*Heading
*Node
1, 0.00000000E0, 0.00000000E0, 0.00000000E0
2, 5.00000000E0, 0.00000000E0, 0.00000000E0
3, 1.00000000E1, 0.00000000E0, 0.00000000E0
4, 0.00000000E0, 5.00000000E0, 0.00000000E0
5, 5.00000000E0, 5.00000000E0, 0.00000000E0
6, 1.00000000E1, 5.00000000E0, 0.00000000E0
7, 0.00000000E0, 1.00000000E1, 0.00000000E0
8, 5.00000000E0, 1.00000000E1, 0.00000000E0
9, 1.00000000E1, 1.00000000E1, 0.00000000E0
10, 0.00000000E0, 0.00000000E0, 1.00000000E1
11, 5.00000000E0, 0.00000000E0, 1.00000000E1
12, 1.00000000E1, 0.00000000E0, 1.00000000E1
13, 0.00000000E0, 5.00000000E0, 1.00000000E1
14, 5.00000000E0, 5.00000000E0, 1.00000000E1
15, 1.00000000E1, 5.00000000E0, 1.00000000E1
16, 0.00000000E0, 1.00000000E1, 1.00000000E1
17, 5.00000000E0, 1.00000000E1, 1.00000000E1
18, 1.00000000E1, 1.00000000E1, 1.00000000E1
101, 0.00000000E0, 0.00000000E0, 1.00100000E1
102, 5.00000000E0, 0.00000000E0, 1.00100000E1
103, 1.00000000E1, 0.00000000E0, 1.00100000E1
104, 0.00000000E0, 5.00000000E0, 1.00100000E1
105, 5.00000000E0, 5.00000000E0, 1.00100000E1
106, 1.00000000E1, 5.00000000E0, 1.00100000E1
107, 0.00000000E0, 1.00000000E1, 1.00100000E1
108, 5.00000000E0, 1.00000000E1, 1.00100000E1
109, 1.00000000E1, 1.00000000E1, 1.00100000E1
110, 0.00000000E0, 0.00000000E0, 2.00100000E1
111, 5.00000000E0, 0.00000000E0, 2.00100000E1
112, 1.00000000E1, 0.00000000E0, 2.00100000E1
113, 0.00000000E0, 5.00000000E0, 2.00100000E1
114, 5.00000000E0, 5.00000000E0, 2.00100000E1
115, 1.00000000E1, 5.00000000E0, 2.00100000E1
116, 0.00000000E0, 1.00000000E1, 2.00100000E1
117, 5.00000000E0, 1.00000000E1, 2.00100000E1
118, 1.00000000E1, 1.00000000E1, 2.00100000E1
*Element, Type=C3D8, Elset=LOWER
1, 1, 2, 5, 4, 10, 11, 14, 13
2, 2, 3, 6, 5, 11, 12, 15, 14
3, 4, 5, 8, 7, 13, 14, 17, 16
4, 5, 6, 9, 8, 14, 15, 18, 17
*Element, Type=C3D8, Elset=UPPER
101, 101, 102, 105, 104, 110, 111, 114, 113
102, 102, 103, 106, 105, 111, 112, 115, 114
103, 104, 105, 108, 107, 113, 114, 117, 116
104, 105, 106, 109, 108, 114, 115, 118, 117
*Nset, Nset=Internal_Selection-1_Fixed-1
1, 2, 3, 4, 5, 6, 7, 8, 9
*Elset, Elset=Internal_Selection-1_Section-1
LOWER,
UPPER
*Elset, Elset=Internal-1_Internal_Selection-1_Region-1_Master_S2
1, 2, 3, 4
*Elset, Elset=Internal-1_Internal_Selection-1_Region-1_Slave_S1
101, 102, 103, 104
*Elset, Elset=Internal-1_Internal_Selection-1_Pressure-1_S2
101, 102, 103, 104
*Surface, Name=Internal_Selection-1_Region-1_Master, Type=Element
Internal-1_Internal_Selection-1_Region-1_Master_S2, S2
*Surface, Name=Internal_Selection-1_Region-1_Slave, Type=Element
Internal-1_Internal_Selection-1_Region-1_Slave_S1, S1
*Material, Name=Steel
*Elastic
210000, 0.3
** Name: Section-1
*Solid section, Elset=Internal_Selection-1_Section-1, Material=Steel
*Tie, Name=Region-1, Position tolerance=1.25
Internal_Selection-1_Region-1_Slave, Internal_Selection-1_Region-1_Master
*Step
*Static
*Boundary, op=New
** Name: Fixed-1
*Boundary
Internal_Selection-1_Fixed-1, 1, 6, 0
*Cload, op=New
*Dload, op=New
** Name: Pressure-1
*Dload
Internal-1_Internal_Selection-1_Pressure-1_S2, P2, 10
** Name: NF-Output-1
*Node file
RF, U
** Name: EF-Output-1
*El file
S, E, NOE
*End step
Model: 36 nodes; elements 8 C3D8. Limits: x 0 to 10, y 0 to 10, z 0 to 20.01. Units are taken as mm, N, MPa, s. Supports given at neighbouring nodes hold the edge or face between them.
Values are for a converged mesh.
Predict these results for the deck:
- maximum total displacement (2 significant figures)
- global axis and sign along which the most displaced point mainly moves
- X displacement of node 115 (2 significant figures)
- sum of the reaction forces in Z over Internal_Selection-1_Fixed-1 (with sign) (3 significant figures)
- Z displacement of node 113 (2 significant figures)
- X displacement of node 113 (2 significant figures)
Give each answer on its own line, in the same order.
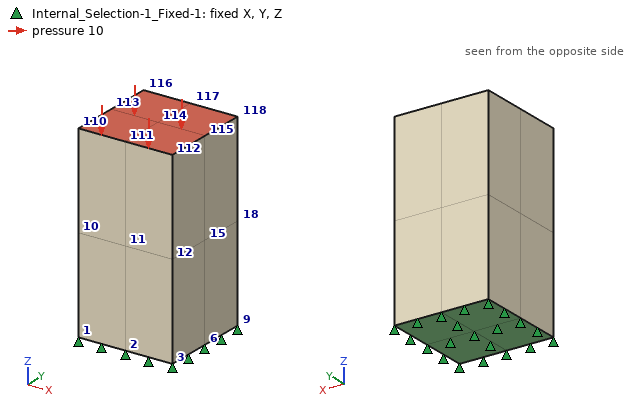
9.3e-04 mm
-Z
7.2e-05 mm
1000 N
-9.3e-04 mm
-7.2e-05 mm
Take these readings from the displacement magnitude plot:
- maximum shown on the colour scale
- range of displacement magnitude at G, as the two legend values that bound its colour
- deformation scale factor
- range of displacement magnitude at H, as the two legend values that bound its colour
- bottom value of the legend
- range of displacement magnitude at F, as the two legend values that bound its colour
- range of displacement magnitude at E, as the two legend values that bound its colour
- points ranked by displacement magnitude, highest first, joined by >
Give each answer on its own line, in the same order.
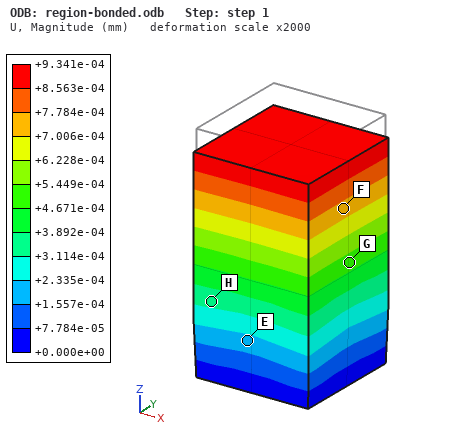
+9.341e-04 mm
+4.671e-04 to +5.449e-04 mm
2000
+3.114e-04 to +3.892e-04 mm
+0.000e+00 mm
+7.006e-04 to +7.784e-04 mm
+1.557e-04 to +2.335e-04 mm
F > G > H > E
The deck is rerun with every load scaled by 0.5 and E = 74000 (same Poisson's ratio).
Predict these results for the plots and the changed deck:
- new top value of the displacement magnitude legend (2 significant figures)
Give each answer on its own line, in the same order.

0.0013 mm
